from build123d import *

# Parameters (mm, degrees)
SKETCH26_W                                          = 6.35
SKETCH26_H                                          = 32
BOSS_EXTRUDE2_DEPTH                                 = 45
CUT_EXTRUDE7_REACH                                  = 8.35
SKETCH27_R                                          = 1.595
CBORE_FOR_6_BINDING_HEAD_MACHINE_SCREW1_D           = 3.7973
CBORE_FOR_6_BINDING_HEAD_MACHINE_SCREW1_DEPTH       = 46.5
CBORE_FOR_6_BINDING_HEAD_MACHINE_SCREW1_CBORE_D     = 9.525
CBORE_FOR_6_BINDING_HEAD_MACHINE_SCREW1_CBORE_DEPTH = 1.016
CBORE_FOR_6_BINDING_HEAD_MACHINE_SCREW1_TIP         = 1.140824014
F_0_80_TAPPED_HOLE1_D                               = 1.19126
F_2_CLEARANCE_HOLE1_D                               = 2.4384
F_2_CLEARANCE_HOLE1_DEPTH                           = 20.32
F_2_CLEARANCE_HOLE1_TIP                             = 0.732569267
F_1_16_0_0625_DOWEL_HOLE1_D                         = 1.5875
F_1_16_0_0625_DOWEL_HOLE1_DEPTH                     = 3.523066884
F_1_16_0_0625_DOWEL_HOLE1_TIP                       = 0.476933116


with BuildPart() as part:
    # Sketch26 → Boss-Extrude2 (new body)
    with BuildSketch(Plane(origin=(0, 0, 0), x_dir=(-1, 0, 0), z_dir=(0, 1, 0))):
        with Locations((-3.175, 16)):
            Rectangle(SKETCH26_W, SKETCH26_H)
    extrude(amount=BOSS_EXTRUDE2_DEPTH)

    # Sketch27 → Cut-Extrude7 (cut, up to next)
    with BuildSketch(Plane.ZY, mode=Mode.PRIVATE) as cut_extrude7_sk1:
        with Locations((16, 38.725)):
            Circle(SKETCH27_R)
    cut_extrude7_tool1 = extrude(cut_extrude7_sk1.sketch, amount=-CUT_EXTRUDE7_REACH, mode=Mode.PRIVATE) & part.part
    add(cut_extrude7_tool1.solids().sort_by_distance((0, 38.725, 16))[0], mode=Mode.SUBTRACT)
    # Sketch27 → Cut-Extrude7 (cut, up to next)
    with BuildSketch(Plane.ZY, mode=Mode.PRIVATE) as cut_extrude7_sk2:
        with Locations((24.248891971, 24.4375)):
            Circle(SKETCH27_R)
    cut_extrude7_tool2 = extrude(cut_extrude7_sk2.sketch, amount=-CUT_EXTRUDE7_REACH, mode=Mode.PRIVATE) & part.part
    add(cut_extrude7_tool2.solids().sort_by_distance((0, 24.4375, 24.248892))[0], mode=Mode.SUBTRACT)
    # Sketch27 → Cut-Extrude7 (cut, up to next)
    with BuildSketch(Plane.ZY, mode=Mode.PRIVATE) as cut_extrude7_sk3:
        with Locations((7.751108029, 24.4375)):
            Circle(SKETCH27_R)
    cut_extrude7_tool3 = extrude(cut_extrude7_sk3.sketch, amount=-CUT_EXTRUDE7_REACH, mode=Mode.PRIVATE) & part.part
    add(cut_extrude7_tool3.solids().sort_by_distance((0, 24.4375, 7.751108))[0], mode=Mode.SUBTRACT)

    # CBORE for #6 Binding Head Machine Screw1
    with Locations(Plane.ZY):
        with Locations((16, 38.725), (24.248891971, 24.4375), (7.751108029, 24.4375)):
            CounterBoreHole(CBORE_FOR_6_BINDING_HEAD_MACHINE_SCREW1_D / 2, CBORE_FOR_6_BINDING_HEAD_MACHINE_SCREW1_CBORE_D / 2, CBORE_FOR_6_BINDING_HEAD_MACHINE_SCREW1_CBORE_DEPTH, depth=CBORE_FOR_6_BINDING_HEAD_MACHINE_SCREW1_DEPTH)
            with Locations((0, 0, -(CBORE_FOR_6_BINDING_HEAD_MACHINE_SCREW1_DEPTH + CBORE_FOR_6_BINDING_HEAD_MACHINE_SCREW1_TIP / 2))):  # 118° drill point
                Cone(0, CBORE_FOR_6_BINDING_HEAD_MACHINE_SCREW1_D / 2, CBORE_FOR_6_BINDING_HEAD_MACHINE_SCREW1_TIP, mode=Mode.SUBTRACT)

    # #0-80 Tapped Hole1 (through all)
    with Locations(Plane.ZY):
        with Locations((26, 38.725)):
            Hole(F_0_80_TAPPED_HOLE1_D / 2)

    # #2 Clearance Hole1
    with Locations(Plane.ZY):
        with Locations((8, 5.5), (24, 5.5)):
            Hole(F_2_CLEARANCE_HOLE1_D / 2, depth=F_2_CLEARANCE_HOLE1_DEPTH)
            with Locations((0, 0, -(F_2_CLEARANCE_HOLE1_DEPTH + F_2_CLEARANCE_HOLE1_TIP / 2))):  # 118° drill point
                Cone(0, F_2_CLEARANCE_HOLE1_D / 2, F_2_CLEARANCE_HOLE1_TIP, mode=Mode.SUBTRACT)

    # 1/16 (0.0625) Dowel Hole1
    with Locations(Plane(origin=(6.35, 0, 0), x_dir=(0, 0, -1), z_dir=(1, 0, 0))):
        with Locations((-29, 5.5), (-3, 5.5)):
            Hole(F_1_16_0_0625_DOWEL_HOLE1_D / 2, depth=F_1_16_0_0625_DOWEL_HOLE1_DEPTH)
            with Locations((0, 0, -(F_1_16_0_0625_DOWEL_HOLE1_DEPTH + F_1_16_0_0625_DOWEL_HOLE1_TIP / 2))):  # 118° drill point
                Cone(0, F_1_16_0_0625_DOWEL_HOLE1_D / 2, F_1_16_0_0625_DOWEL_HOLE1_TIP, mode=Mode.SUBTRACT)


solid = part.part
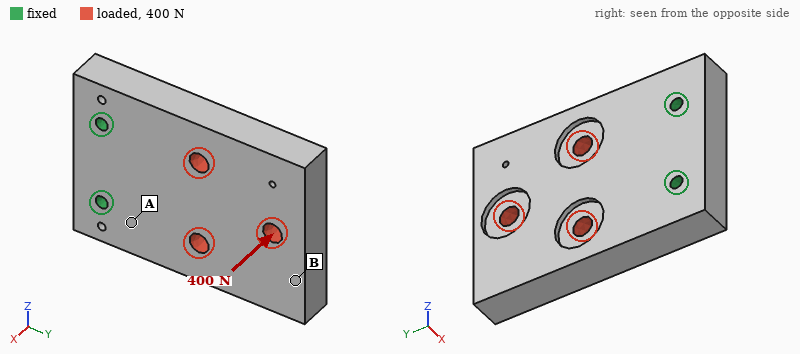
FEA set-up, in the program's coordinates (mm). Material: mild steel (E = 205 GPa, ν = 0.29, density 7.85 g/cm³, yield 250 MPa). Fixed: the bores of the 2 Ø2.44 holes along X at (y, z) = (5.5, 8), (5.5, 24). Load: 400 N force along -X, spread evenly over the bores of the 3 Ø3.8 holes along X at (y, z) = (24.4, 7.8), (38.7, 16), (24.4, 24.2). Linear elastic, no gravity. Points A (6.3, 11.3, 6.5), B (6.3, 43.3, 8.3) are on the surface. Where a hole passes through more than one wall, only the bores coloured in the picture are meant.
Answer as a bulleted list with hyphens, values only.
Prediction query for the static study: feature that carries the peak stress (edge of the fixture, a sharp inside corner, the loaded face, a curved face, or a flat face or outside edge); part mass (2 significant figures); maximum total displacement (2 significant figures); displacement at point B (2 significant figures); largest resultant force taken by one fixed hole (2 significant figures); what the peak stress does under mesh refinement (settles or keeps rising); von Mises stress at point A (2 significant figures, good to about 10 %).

- edge of the fixture
- 68 g
- 34 µm
- 32 µm
- 200 N
- keeps rising
- 34 MPa
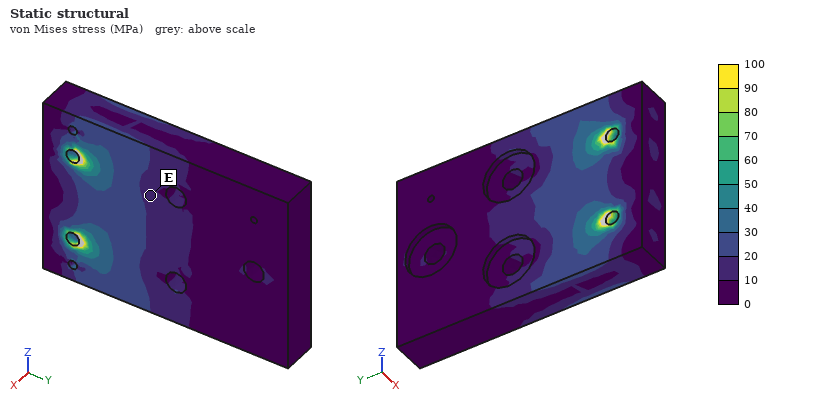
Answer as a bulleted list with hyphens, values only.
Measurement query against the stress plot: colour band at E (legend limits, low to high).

- 10 to 20 MPa
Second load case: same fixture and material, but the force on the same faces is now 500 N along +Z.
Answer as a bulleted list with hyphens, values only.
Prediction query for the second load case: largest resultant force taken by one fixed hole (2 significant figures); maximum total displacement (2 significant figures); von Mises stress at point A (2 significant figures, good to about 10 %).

- 720 N
- 3.9 µm
- 7.7 MPa
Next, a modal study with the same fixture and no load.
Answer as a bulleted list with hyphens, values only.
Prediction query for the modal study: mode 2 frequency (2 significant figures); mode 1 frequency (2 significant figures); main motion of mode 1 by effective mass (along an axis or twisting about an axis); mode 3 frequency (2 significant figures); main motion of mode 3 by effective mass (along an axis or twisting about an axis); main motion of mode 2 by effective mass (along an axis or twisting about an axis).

- 7900 Hz
- 3100 Hz
- along X
- 9600 Hz
- along Z
- twisting about Y
